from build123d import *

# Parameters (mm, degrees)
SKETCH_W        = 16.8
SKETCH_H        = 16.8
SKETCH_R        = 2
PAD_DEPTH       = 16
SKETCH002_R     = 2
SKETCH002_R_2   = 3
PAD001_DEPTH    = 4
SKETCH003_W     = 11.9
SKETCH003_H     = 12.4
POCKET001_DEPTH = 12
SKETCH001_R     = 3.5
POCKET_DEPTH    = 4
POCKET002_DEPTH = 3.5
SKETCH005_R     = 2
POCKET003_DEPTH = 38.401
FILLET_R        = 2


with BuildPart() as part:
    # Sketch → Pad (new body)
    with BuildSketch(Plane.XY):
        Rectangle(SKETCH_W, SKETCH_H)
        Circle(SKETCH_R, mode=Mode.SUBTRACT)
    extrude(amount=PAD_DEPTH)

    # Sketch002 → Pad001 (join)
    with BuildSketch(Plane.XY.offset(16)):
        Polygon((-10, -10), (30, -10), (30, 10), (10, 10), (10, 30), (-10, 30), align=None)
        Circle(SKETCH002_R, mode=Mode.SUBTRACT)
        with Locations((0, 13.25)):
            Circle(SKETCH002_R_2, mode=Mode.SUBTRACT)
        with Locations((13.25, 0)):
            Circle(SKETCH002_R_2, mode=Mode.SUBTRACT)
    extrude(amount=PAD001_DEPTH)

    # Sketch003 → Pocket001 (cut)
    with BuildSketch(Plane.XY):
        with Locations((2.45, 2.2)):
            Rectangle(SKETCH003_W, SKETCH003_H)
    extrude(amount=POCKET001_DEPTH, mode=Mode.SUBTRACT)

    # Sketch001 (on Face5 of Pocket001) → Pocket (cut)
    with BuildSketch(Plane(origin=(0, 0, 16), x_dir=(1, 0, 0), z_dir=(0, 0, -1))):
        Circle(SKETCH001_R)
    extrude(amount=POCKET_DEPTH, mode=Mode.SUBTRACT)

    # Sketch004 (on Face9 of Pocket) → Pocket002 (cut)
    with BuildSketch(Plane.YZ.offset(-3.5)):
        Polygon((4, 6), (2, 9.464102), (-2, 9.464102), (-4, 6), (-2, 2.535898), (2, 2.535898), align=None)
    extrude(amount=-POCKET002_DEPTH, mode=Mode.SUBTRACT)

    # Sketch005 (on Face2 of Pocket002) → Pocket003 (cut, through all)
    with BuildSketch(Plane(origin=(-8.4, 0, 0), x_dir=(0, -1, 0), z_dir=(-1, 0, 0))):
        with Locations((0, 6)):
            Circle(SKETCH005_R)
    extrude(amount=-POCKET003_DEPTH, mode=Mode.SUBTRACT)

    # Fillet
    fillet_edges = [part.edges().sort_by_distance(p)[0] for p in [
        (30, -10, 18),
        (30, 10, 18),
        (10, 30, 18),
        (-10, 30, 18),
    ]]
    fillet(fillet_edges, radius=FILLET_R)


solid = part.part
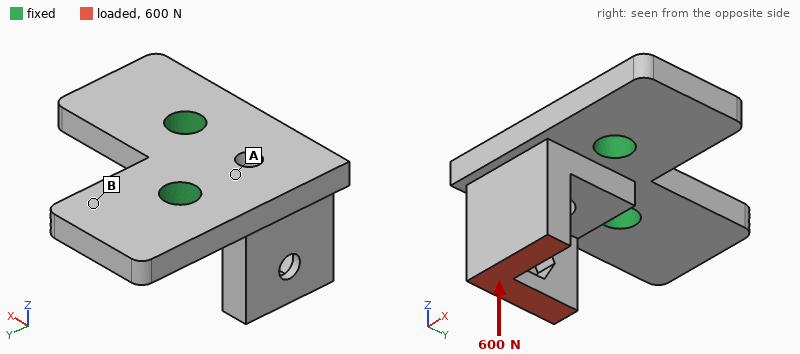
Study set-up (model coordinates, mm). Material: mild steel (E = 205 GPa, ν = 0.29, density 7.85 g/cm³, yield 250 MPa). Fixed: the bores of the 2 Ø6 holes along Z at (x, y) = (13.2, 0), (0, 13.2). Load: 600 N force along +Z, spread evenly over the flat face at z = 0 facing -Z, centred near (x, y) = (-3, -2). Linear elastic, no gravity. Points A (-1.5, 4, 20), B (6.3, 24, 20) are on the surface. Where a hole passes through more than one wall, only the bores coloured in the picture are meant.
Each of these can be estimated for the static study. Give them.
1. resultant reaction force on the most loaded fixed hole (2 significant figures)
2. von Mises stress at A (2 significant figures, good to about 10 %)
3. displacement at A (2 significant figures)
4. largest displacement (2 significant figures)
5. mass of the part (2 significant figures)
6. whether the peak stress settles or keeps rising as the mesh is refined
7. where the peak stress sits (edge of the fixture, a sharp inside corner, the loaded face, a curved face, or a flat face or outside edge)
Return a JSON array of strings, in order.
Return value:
["310 N", "21 MPa", "3.4 µm", "19 µm", "54 g", "keeps rising", "edge of the fixture"]
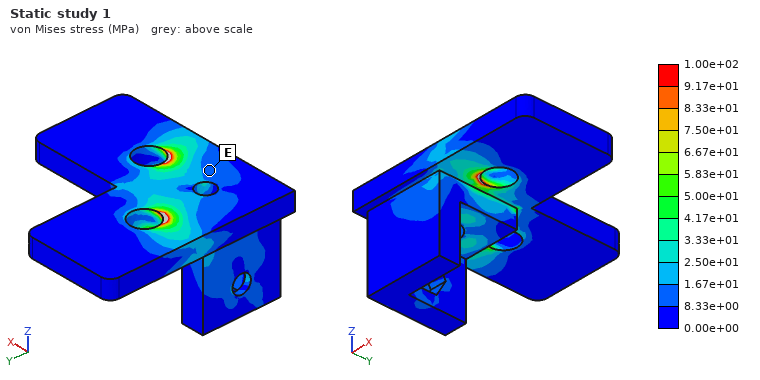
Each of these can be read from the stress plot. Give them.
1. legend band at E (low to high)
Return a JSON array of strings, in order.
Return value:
["8.33e+00 to 1.67e+01 MPa"]
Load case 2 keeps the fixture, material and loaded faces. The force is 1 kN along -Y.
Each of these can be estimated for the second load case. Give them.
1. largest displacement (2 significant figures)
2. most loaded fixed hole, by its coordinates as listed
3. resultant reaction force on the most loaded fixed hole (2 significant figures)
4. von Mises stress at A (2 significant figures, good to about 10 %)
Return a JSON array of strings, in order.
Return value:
["54 µm", "(0, 13.2)", "1.1 kN", "68 MPa"]
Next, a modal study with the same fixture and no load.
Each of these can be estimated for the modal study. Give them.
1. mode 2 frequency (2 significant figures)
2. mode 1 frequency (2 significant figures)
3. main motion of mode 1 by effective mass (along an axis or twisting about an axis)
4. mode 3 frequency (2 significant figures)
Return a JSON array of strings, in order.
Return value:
["13 kHz", "6600 Hz", "along Z", "13 kHz"]
